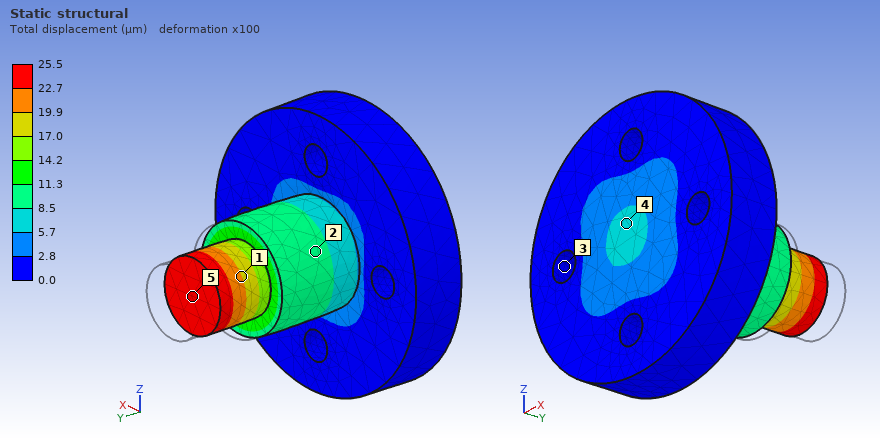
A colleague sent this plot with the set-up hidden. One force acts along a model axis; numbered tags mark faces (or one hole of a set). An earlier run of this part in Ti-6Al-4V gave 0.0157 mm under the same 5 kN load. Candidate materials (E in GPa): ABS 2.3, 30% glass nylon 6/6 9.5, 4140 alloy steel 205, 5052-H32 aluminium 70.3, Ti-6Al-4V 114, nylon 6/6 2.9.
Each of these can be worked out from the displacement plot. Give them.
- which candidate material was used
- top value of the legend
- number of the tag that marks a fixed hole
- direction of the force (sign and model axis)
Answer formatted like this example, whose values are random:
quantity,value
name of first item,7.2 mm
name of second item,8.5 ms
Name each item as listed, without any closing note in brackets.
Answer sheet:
quantity,value
which candidate material was used,5052-H32 aluminium
top value of the legend,25.5 µm
number of the tag that marks a fixed hole,3
direction of the force,-Y
